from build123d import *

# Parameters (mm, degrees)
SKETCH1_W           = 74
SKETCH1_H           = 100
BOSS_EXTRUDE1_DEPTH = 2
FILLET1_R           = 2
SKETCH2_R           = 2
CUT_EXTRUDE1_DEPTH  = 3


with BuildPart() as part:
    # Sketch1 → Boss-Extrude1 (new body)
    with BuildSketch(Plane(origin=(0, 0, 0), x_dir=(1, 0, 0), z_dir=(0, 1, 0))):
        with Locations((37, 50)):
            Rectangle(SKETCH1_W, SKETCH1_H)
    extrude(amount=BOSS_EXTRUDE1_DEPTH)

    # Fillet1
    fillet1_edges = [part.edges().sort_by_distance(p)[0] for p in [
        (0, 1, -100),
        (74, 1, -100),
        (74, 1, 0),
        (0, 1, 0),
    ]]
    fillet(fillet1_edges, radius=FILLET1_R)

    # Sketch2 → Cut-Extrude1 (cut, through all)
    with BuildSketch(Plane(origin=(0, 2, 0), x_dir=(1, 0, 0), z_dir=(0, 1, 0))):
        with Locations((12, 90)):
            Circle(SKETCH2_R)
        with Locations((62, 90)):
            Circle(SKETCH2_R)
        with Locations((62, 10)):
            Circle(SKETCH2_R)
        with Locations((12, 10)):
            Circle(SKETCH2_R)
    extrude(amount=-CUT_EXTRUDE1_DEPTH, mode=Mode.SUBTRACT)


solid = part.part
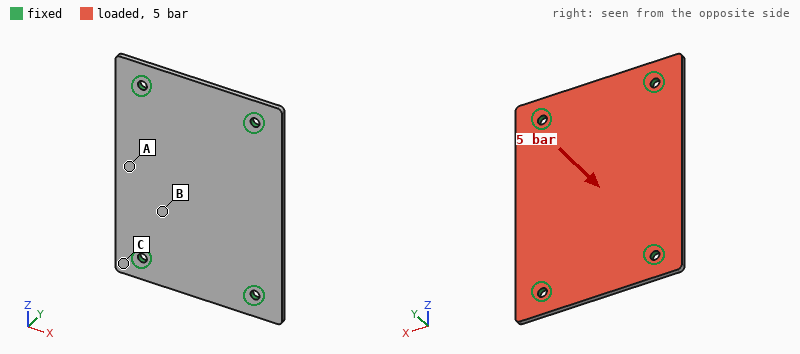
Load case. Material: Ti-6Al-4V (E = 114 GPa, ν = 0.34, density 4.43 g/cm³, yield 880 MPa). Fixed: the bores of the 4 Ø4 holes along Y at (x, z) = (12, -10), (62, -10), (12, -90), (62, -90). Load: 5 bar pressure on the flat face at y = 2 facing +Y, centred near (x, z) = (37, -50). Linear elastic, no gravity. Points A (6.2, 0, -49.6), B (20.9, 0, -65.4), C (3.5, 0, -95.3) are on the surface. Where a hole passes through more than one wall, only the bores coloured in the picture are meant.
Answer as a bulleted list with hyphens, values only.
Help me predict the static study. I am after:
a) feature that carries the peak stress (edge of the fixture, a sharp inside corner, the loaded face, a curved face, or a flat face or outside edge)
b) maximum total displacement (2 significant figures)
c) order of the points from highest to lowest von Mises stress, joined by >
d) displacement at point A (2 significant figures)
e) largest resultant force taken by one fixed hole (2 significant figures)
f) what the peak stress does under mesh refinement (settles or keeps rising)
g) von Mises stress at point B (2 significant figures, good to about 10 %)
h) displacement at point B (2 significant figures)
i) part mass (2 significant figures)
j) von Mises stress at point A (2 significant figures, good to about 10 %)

- edge of the fixture
- 0.86 mm
- A > B > C
- 0.79 mm
- 920 N
- keeps rising
- 130 MPa
- 0.63 mm
- 65 g
- 220 MPa
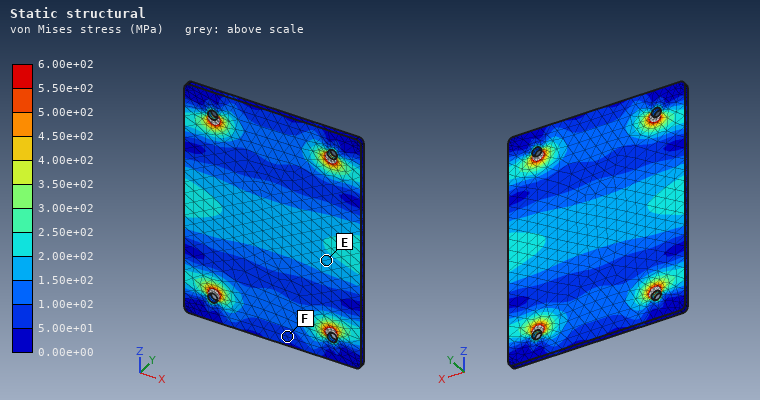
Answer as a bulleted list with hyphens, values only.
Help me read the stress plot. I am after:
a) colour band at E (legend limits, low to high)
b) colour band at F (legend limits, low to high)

- 1.50e+02 to 2.00e+02 MPa
- 5.00e+01 to 1.00e+02 MPa
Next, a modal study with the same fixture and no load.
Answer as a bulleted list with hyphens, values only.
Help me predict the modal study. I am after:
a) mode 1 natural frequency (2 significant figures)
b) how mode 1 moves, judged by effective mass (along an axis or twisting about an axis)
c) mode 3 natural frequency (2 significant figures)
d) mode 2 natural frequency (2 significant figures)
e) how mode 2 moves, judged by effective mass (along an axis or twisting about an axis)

- 1500 Hz
- along Y
- 3100 Hz
- 2000 Hz
- twisting about Z
